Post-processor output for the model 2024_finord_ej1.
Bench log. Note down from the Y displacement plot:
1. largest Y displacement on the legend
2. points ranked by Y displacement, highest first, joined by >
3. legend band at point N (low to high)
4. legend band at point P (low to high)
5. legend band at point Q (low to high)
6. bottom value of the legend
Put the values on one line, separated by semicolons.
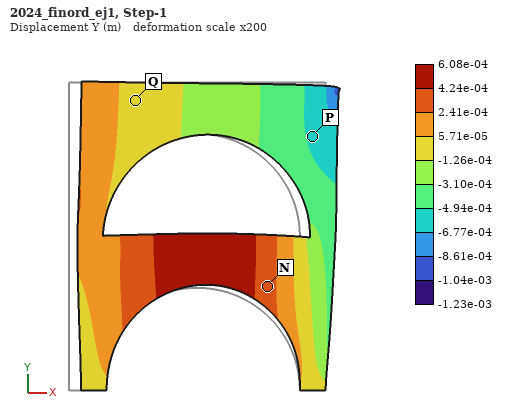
6.08e-04 m; N > Q > P; 2.41e-04 to 4.24e-04 m; -6.77e-04 to -4.94e-04 m; -1.26e-04 to 5.71e-05 m; -1.23e-03 m
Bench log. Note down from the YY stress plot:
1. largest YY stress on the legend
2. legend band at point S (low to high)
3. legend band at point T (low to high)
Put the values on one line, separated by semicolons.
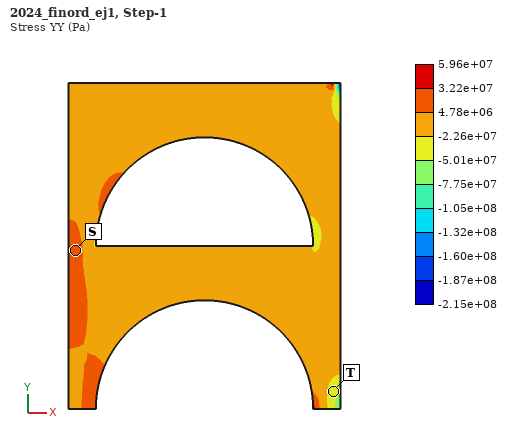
5.96e+07 Pa; 4.78e+06 to 3.22e+07 Pa; -5.01e+07 to -2.26e+07 Pa
